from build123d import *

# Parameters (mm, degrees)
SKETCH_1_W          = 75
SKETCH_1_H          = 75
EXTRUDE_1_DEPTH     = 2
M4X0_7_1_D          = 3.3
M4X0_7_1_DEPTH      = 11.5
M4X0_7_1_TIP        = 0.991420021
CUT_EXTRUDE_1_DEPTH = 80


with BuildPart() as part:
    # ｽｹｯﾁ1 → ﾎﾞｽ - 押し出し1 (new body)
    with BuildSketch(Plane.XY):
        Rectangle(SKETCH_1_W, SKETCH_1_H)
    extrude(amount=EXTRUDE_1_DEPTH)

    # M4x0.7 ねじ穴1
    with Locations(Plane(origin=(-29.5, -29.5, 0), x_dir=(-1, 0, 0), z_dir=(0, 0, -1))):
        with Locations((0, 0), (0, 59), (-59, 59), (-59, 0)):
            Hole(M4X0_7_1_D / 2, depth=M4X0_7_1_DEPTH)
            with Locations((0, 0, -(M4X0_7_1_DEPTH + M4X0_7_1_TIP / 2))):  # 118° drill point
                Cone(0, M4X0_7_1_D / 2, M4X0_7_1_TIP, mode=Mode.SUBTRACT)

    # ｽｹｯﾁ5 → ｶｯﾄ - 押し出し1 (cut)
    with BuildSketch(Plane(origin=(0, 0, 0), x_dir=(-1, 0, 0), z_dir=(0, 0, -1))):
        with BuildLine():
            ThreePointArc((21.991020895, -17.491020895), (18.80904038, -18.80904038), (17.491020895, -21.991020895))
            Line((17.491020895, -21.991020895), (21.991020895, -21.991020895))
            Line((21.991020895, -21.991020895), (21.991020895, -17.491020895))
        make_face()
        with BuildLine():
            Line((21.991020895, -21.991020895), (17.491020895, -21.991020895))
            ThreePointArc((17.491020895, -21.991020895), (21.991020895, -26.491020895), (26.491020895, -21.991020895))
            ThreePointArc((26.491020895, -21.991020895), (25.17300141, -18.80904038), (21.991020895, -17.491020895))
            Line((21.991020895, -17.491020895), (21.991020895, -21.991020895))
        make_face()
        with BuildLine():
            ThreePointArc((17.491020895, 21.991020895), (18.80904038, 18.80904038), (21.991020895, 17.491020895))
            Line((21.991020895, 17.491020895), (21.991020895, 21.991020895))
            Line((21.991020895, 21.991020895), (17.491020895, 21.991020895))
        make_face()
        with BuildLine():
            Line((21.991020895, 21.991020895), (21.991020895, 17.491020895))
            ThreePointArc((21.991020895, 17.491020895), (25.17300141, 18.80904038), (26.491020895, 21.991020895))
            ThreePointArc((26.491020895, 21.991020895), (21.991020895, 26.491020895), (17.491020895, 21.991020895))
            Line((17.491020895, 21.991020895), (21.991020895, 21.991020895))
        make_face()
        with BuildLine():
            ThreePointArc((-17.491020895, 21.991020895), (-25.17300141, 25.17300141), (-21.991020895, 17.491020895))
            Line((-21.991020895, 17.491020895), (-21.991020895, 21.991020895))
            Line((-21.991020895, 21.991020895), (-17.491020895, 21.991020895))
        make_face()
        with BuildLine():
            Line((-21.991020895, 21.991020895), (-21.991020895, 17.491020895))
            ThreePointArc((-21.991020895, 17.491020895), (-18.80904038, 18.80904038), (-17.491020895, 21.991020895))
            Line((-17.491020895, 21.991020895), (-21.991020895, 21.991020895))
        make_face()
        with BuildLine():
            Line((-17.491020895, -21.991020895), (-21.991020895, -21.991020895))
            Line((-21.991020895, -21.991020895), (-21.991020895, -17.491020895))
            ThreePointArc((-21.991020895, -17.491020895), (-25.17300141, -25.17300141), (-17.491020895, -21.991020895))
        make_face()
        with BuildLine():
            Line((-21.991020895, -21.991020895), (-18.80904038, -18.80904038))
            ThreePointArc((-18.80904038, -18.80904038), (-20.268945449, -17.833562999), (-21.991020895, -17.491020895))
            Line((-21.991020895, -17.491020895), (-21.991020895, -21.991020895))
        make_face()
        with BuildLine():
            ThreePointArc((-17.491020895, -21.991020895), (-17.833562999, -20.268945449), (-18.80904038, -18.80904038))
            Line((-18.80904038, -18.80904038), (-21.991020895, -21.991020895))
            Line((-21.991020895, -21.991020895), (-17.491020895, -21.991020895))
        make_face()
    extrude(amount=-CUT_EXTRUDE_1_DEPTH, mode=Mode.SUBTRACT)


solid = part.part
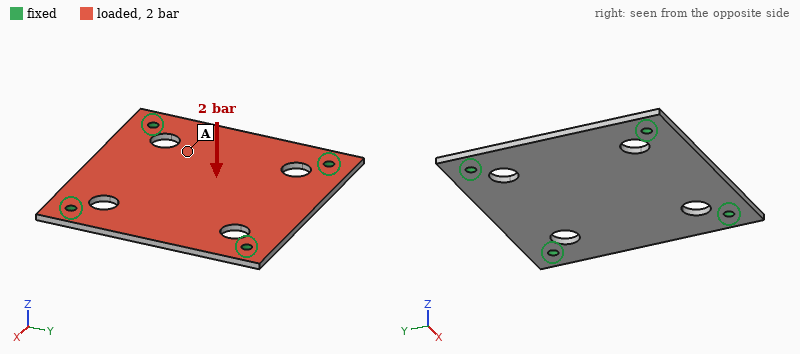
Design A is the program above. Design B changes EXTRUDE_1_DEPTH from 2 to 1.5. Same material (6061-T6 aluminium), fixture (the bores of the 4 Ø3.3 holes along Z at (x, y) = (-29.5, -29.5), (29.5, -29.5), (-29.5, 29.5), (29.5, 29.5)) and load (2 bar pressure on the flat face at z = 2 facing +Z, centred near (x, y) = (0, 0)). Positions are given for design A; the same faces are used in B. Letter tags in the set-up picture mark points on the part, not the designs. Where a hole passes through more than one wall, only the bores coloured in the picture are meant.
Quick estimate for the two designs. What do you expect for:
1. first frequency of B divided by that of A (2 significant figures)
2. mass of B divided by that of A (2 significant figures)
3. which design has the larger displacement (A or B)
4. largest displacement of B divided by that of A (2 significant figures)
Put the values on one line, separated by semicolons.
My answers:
0.76; 0.75; B; 2.3
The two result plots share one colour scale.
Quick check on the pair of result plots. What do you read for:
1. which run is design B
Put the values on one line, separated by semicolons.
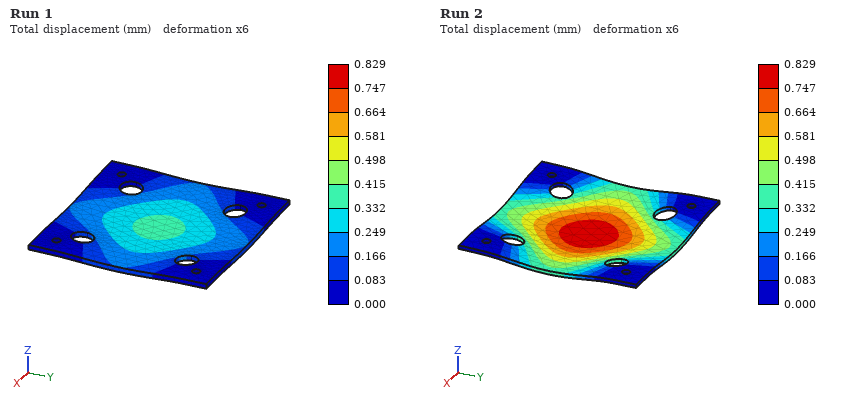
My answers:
Run 2
